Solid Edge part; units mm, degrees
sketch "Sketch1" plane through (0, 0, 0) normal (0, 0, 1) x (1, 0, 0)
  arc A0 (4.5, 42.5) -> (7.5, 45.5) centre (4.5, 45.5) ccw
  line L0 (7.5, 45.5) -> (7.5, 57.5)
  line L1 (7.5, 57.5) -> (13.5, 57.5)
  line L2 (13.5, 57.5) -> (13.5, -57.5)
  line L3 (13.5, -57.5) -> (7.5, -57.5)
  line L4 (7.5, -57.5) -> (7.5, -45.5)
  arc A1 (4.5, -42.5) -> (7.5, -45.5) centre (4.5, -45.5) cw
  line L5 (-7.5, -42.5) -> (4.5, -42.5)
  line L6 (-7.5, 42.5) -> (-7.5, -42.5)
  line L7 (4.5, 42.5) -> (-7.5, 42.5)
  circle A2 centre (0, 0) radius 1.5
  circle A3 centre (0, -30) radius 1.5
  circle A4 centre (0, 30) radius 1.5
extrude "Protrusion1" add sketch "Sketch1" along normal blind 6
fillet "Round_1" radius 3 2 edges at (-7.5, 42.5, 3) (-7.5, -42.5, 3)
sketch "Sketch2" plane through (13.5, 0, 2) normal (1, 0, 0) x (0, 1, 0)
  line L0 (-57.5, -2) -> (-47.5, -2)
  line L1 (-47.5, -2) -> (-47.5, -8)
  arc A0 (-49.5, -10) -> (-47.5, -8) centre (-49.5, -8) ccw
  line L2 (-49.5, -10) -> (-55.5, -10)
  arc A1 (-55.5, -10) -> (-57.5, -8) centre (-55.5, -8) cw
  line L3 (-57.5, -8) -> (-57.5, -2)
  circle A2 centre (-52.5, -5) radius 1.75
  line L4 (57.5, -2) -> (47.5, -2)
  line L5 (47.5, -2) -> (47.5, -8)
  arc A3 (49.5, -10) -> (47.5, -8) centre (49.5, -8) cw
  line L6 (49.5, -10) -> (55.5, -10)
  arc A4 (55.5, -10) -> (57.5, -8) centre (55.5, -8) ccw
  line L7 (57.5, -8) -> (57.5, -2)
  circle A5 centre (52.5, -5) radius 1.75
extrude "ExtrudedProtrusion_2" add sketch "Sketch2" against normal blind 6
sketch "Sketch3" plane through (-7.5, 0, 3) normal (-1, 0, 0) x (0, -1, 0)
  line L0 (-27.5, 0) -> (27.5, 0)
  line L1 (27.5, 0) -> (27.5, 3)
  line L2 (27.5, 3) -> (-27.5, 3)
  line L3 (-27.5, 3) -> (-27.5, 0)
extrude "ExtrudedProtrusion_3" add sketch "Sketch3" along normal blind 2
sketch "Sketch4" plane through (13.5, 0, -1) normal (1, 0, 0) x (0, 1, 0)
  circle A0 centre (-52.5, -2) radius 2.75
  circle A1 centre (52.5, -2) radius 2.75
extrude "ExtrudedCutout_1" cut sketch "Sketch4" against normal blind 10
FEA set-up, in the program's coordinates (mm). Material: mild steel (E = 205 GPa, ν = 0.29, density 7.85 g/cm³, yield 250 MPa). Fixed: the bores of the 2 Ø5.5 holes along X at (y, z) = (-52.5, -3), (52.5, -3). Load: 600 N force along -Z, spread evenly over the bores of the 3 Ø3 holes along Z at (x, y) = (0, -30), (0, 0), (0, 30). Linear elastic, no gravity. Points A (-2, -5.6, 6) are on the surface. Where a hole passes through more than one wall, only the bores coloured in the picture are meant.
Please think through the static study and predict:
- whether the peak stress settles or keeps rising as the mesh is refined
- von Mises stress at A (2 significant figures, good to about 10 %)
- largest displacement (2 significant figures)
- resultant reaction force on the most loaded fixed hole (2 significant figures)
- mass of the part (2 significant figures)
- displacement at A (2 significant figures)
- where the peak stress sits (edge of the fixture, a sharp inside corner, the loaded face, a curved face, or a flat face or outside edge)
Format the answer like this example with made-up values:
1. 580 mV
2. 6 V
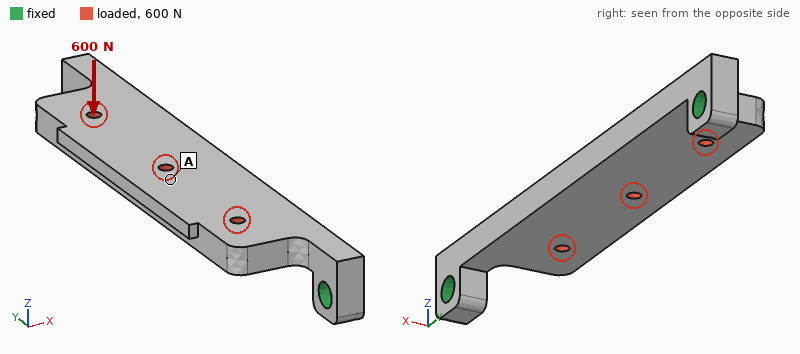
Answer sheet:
1. keeps rising
2. 29 MPa
3. 92 µm
4. 370 N
5. 99 g
6. 73 µm
7. a sharp inside corner
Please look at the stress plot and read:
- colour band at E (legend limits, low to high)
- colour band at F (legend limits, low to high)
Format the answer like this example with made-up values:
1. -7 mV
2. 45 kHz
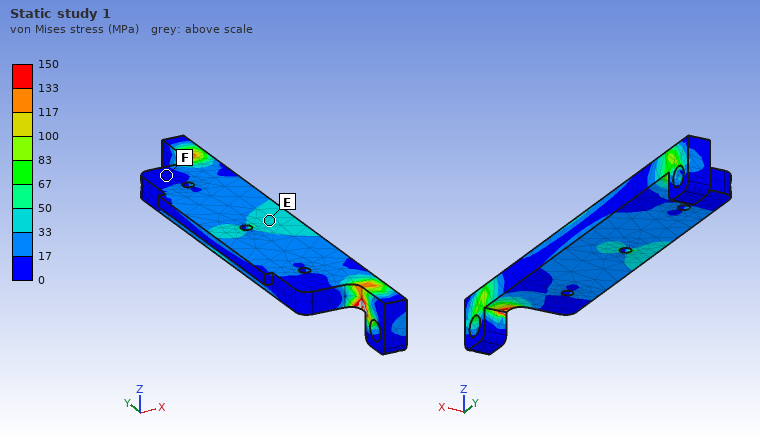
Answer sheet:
1. 33 to 50 MPa
2. 0 to 17 MPa
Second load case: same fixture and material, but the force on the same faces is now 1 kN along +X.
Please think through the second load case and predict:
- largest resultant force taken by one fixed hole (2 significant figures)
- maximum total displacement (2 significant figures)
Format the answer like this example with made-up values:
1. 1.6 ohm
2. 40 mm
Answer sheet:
1. 680 N
2. 16 µm
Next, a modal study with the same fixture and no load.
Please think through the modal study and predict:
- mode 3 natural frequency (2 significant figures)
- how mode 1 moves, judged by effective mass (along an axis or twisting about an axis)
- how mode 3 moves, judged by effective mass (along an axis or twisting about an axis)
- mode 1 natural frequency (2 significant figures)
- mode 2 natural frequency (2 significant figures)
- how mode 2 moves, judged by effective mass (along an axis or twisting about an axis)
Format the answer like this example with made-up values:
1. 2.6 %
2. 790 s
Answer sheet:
1. 5200 Hz
2. along Z
3. along X
4. 1900 Hz
5. 4400 Hz
6. twisting about Y
